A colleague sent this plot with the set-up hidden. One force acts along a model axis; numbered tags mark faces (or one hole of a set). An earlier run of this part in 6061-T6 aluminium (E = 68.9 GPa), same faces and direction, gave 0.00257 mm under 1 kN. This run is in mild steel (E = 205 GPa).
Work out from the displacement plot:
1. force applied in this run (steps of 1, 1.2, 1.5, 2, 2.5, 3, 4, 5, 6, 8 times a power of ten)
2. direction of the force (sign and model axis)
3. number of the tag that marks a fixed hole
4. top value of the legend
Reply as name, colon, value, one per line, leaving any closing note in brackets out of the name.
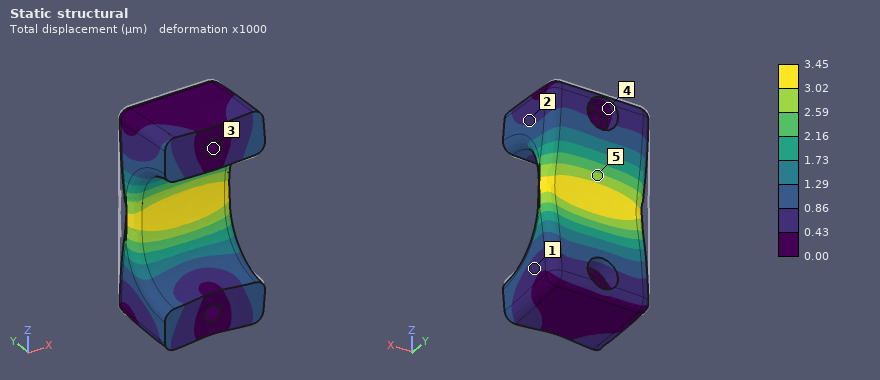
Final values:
force applied in this run: 4 kN
direction of the force: -Y
number of the tag that marks a fixed hole: 3
top value of the legend: 3.45 µm
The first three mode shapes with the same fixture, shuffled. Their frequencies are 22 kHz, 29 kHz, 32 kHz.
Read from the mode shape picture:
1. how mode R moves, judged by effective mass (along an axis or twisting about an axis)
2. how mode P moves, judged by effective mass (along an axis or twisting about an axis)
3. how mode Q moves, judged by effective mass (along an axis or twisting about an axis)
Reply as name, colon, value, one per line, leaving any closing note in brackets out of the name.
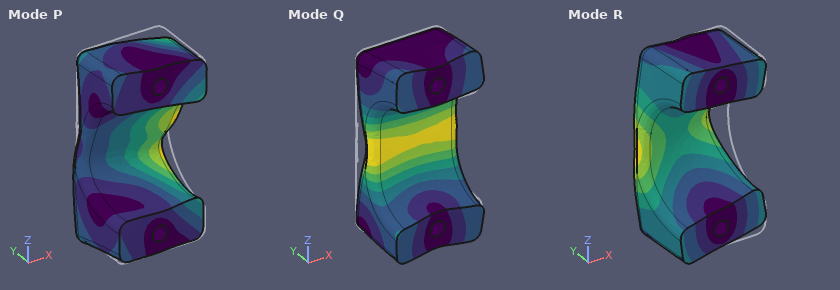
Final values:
how mode R moves, judged by effective mass: along X
how mode P moves, judged by effective mass: along Z
how mode Q moves, judged by effective mass: along Y
